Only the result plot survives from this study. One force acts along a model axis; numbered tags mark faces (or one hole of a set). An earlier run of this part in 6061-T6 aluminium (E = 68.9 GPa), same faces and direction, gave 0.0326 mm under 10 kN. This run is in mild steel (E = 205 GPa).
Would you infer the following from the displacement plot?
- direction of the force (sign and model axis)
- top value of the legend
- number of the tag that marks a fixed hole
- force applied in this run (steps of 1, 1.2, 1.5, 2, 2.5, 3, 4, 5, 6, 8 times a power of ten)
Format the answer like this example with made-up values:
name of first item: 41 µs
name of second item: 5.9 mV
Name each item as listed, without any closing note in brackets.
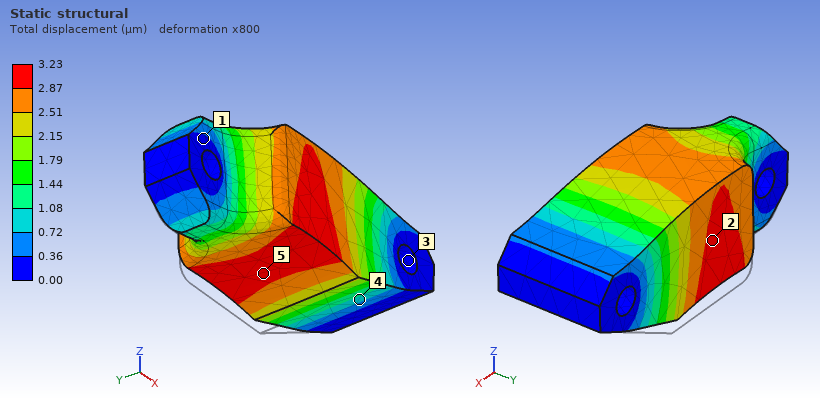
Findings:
direction of the force: +Z
top value of the legend: 3.23 µm
number of the tag that marks a fixed hole: 3
force applied in this run: 3 kN
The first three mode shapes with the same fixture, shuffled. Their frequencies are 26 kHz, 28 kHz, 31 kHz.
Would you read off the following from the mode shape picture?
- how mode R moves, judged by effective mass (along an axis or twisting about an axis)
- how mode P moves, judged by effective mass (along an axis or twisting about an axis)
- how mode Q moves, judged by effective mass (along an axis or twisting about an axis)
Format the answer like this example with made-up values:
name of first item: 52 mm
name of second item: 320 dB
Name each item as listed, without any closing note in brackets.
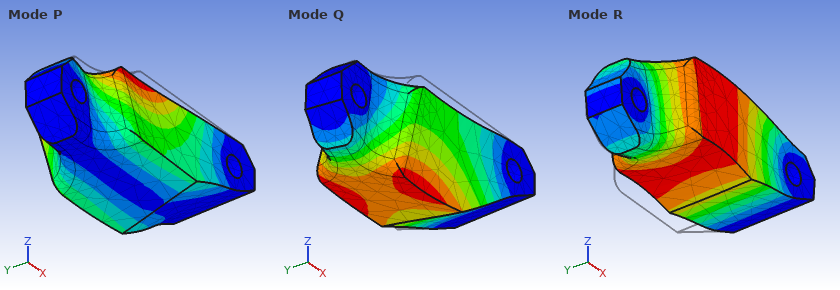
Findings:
how mode R moves, judged by effective mass: along Z
how mode P moves, judged by effective mass: along Y
how mode Q moves, judged by effective mass: along Y
